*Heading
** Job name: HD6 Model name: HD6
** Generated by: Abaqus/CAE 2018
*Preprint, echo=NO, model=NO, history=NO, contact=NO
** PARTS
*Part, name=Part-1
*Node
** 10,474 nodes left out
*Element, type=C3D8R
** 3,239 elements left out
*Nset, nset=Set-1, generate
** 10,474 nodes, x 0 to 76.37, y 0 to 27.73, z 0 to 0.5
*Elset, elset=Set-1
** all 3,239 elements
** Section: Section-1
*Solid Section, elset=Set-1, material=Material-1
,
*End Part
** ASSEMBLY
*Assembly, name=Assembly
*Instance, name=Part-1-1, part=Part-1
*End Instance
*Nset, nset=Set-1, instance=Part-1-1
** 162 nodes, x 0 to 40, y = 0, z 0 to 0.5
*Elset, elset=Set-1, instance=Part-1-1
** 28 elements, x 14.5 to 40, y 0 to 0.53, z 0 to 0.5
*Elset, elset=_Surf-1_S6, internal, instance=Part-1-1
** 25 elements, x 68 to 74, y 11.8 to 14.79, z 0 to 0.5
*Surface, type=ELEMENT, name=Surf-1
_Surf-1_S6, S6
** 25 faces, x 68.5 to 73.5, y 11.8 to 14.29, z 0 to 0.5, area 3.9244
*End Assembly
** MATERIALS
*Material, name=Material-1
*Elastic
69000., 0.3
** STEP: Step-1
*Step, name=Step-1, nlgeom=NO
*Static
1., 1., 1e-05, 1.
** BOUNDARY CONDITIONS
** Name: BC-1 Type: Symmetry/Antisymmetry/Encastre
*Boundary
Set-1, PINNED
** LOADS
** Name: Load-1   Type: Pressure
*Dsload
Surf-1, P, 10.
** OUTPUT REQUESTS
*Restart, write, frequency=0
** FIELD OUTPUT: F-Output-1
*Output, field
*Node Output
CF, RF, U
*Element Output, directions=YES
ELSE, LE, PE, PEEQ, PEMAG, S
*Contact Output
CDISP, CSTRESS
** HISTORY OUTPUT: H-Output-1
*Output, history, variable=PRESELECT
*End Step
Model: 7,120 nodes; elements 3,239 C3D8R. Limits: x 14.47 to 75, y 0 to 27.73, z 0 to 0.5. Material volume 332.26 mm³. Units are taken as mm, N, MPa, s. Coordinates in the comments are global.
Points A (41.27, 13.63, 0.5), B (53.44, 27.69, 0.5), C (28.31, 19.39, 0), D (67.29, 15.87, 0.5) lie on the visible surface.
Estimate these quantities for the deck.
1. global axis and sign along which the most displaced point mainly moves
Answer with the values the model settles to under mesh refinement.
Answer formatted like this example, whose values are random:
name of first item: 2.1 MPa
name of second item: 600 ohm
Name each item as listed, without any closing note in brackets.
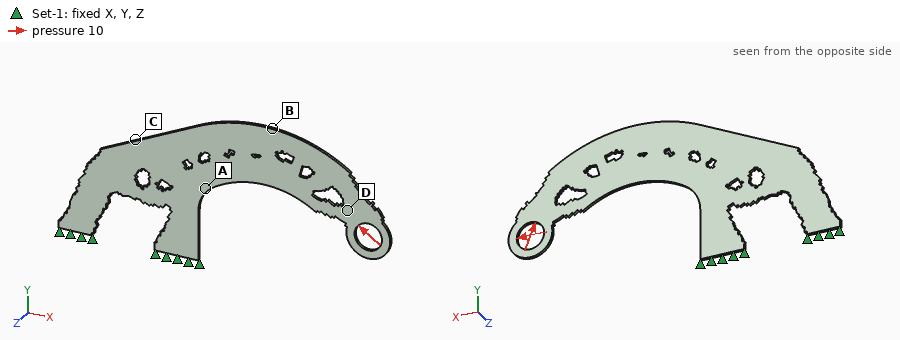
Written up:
global axis and sign along which the most displaced point mainly moves: +Y
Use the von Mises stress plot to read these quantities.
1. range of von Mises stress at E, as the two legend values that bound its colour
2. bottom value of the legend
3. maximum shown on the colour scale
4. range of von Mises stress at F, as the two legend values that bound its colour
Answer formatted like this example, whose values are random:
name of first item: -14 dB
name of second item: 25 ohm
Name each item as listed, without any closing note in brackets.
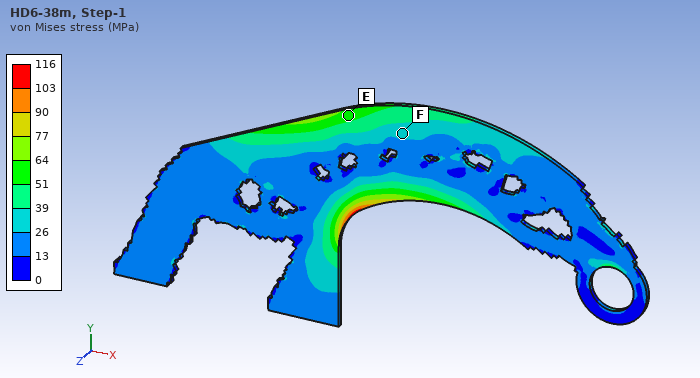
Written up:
range of von Mises stress at E, as the two legend values that bound its colour: 51 to 64 MPa
bottom value of the legend: 0 MPa
maximum shown on the colour scale: 116 MPa
range of von Mises stress at F, as the two legend values that bound its colour: 26 to 39 MPa
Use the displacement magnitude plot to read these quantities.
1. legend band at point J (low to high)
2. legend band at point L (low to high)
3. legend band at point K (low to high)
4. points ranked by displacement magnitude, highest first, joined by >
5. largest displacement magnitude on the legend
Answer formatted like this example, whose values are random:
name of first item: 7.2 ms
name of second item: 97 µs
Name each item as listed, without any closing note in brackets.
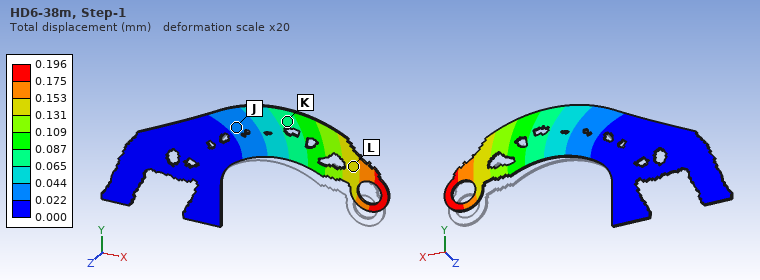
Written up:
legend band at point J: 0.022 to 0.044 mm
legend band at point L: 0.131 to 0.153 mm
legend band at point K: 0.065 to 0.087 mm
points ranked by displacement magnitude, highest first, joined by >: L > K > J
largest displacement magnitude on the legend: 0.196 mm
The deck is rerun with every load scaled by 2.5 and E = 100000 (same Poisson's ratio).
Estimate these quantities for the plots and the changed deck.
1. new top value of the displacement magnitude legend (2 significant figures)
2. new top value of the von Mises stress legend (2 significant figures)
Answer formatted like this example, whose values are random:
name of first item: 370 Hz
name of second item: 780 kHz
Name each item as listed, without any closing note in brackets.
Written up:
new top value of the displacement magnitude legend: 0.34 mm
new top value of the von Mises stress legend: 290 MPa
